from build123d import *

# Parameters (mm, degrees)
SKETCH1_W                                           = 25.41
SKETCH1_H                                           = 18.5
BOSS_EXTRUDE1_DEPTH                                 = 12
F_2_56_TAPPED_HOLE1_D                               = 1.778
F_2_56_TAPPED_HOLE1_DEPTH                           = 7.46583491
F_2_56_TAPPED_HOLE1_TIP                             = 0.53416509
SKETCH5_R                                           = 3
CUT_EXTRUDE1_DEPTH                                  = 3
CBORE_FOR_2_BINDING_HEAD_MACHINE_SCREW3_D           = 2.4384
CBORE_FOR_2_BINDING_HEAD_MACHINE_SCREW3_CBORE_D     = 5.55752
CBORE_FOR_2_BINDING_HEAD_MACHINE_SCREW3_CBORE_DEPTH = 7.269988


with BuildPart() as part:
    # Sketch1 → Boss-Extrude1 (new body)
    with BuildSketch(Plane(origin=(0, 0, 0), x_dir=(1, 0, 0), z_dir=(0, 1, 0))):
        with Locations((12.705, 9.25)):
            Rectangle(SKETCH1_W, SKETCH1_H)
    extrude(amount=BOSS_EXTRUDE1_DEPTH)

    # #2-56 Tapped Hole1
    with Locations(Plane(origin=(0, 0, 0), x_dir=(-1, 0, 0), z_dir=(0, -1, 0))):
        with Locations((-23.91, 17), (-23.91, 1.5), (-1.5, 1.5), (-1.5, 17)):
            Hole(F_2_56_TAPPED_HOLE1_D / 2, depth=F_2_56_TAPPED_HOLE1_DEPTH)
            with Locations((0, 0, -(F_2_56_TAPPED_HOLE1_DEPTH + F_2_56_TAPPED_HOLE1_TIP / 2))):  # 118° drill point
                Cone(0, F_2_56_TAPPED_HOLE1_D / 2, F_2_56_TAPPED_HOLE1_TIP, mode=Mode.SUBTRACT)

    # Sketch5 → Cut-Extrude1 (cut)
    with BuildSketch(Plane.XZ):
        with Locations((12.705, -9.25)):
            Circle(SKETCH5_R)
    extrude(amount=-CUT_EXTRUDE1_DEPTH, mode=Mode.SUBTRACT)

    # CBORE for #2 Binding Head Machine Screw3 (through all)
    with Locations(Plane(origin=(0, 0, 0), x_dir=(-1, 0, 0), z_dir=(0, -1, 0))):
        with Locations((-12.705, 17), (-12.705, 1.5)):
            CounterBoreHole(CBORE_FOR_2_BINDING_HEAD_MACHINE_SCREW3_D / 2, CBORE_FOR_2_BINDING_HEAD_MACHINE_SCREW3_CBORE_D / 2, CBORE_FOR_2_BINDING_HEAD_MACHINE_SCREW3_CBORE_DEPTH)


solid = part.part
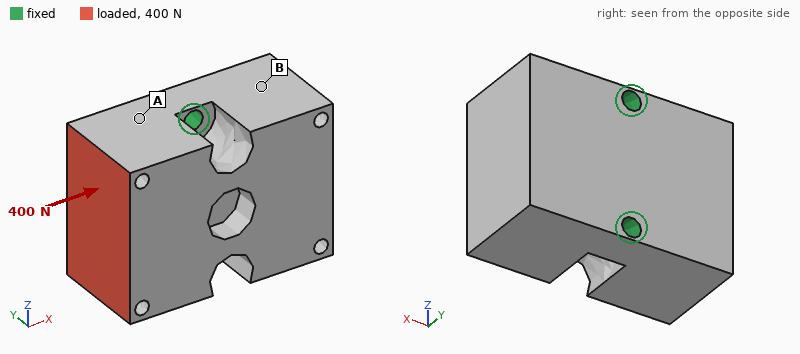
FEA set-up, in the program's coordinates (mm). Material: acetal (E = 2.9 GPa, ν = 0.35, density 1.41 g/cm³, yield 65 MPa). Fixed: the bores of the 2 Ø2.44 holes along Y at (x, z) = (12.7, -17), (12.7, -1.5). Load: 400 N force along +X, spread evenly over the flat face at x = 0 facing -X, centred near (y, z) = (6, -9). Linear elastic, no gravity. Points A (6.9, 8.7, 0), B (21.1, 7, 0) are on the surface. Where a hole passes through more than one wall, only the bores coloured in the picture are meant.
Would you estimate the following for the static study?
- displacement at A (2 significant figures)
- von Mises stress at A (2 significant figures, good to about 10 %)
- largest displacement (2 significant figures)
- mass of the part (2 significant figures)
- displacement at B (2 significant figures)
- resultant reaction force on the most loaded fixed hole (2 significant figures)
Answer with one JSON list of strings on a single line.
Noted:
["0.039 mm", "6.0 MPa", "0.13 mm", "7.3 g", "0.059 mm", "200 N"]
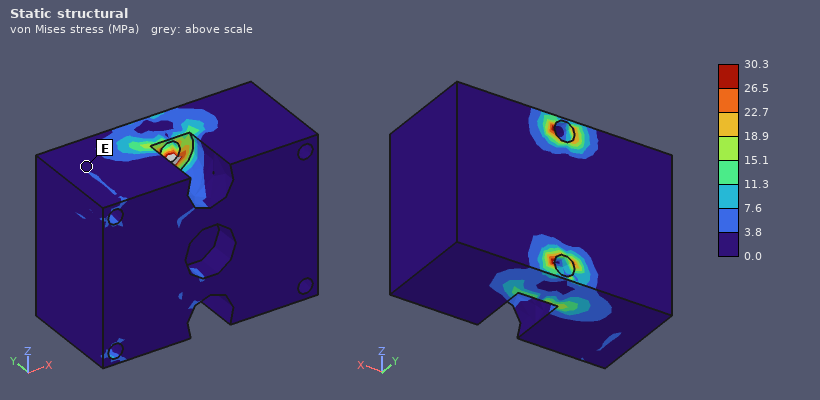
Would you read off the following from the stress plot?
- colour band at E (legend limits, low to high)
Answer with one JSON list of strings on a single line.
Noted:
["0.0 to 3.8 MPa"]
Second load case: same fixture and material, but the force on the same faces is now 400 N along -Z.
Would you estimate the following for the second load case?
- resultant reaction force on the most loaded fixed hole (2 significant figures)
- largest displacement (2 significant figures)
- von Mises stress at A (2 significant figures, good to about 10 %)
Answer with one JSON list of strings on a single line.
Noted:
["390 N", "87 µm", "7.1 MPa"]
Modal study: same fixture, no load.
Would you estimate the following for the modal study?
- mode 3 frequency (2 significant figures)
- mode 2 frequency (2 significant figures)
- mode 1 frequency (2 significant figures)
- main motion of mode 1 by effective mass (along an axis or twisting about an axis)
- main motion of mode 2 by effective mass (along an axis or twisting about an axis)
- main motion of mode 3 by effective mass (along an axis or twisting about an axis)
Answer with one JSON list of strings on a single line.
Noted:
["8200 Hz", "7800 Hz", "3000 Hz", "along X", "along Y", "along Z"]
